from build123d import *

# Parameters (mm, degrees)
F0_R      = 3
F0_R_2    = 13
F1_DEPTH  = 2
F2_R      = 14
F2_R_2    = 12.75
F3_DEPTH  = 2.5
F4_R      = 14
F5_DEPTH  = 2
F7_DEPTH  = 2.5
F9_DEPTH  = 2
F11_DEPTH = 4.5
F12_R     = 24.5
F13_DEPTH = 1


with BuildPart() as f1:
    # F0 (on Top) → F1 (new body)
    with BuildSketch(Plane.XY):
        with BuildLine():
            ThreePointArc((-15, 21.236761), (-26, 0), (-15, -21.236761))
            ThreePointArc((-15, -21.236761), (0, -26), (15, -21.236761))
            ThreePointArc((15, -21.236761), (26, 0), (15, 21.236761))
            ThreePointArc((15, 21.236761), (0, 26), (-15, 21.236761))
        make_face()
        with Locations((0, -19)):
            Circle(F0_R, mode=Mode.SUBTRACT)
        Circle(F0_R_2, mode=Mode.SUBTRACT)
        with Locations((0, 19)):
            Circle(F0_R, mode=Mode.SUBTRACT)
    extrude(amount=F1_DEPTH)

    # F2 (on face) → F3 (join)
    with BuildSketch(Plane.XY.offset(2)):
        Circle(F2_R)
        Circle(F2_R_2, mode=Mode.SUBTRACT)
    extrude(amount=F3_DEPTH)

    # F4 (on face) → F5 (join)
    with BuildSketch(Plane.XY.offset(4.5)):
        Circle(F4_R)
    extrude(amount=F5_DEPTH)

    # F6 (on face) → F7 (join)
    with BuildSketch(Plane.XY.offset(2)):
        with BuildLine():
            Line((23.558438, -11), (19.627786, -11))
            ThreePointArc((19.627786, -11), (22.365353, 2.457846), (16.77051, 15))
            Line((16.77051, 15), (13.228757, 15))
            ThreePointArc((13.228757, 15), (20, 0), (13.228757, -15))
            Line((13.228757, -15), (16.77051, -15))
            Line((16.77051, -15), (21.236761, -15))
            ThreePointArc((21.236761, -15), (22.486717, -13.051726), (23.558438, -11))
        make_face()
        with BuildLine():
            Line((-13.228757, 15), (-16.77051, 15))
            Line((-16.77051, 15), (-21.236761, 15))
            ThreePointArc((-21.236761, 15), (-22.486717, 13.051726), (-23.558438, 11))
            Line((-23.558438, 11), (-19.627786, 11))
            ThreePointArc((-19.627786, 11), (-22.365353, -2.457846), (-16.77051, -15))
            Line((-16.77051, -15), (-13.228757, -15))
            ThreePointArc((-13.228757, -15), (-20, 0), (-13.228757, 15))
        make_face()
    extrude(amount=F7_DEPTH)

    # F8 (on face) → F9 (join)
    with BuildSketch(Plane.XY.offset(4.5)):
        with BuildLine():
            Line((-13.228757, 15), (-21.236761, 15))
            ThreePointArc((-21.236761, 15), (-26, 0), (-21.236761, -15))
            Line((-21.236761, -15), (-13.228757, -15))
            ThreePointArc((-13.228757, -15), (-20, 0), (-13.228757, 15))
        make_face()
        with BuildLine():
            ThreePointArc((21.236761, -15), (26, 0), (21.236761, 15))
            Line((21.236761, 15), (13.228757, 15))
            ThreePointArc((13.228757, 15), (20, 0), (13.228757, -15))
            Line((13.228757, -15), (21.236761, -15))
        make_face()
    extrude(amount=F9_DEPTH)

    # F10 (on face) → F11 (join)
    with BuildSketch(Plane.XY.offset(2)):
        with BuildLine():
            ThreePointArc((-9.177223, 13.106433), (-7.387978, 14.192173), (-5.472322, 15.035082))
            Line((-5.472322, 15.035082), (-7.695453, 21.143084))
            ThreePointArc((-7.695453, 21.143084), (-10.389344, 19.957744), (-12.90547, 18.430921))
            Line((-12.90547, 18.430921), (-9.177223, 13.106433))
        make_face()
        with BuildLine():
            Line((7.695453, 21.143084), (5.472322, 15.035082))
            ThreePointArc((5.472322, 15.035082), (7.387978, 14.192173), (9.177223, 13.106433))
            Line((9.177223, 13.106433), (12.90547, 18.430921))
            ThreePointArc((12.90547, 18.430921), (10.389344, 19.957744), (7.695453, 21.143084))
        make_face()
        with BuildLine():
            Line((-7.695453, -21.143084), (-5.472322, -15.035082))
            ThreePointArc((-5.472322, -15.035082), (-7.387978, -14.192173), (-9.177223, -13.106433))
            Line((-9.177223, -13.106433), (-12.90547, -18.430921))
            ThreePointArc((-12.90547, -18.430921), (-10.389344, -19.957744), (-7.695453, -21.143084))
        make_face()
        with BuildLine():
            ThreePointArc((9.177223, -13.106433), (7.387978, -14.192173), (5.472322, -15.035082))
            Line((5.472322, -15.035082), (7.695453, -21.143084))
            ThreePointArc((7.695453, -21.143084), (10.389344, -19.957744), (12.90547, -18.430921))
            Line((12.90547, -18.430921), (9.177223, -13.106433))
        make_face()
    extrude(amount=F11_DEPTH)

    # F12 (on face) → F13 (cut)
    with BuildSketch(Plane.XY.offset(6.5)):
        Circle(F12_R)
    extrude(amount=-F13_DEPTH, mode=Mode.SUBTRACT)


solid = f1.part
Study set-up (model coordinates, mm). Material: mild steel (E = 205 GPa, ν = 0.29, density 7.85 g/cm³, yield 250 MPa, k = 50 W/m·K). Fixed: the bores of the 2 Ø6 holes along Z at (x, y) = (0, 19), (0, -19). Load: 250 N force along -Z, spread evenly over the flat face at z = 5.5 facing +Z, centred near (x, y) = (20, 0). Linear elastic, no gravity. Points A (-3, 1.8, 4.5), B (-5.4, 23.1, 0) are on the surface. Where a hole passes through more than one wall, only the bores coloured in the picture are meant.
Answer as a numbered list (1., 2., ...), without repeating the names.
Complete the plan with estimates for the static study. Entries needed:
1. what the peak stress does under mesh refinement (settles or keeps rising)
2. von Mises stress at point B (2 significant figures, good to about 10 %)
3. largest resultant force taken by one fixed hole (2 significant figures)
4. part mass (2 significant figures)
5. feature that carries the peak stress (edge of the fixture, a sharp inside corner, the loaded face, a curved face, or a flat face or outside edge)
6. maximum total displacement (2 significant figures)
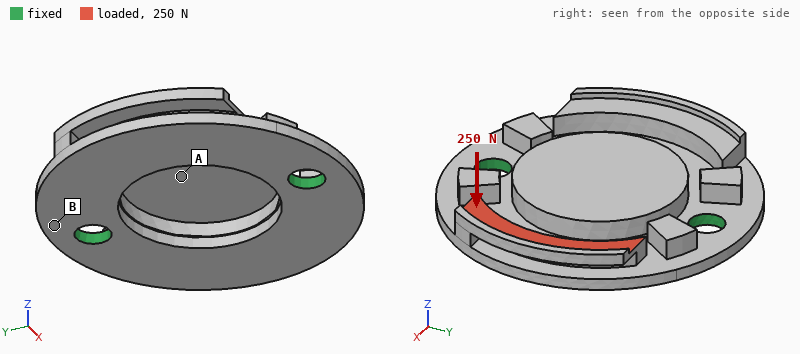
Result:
1. keeps rising
2. 31 MPa
3. 320 N
4. 42 g
5. edge of the fixture
6. 88 µm
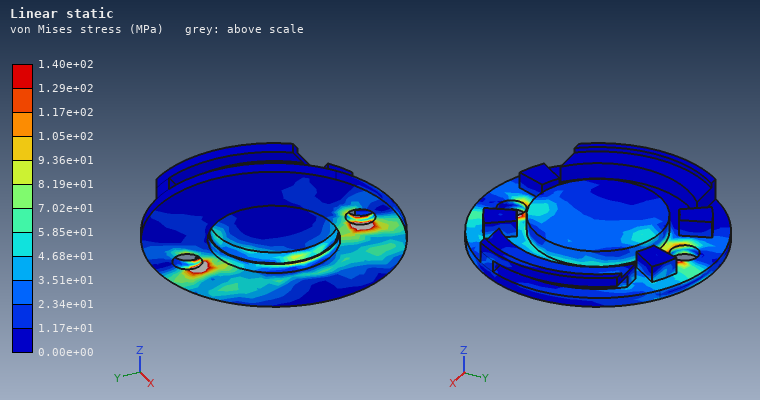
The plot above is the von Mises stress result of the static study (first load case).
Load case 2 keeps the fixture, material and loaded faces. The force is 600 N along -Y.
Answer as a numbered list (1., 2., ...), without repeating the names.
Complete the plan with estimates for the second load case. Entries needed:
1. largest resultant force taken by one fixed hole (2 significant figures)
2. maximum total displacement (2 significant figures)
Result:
1. 410 N
2. 18 µm
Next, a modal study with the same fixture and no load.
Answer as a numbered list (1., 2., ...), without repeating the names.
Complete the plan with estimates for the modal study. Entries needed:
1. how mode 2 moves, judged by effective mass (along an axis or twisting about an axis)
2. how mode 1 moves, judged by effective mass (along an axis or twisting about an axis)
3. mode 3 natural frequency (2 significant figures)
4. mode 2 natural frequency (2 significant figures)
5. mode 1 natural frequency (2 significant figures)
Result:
1. along Z
2. twisting about Y
3. 8100 Hz
4. 4100 Hz
5. 2800 Hz
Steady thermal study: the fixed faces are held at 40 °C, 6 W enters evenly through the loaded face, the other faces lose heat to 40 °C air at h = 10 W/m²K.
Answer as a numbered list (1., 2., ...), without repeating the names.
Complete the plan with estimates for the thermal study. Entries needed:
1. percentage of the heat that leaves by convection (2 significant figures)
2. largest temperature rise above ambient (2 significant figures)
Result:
1. 11 %
2. 37 K
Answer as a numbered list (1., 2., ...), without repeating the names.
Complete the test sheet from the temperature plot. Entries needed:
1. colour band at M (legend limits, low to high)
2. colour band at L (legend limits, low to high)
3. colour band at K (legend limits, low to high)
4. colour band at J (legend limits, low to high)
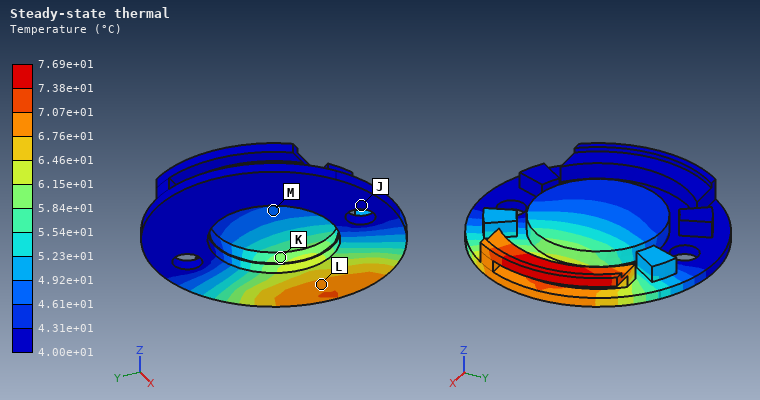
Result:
1. 4.61e+01 to 4.92e+01 °C
2. 6.76e+01 to 7.07e+01 °C
3. 5.84e+01 to 6.15e+01 °C
4. 4.00e+01 to 4.31e+01 °C
